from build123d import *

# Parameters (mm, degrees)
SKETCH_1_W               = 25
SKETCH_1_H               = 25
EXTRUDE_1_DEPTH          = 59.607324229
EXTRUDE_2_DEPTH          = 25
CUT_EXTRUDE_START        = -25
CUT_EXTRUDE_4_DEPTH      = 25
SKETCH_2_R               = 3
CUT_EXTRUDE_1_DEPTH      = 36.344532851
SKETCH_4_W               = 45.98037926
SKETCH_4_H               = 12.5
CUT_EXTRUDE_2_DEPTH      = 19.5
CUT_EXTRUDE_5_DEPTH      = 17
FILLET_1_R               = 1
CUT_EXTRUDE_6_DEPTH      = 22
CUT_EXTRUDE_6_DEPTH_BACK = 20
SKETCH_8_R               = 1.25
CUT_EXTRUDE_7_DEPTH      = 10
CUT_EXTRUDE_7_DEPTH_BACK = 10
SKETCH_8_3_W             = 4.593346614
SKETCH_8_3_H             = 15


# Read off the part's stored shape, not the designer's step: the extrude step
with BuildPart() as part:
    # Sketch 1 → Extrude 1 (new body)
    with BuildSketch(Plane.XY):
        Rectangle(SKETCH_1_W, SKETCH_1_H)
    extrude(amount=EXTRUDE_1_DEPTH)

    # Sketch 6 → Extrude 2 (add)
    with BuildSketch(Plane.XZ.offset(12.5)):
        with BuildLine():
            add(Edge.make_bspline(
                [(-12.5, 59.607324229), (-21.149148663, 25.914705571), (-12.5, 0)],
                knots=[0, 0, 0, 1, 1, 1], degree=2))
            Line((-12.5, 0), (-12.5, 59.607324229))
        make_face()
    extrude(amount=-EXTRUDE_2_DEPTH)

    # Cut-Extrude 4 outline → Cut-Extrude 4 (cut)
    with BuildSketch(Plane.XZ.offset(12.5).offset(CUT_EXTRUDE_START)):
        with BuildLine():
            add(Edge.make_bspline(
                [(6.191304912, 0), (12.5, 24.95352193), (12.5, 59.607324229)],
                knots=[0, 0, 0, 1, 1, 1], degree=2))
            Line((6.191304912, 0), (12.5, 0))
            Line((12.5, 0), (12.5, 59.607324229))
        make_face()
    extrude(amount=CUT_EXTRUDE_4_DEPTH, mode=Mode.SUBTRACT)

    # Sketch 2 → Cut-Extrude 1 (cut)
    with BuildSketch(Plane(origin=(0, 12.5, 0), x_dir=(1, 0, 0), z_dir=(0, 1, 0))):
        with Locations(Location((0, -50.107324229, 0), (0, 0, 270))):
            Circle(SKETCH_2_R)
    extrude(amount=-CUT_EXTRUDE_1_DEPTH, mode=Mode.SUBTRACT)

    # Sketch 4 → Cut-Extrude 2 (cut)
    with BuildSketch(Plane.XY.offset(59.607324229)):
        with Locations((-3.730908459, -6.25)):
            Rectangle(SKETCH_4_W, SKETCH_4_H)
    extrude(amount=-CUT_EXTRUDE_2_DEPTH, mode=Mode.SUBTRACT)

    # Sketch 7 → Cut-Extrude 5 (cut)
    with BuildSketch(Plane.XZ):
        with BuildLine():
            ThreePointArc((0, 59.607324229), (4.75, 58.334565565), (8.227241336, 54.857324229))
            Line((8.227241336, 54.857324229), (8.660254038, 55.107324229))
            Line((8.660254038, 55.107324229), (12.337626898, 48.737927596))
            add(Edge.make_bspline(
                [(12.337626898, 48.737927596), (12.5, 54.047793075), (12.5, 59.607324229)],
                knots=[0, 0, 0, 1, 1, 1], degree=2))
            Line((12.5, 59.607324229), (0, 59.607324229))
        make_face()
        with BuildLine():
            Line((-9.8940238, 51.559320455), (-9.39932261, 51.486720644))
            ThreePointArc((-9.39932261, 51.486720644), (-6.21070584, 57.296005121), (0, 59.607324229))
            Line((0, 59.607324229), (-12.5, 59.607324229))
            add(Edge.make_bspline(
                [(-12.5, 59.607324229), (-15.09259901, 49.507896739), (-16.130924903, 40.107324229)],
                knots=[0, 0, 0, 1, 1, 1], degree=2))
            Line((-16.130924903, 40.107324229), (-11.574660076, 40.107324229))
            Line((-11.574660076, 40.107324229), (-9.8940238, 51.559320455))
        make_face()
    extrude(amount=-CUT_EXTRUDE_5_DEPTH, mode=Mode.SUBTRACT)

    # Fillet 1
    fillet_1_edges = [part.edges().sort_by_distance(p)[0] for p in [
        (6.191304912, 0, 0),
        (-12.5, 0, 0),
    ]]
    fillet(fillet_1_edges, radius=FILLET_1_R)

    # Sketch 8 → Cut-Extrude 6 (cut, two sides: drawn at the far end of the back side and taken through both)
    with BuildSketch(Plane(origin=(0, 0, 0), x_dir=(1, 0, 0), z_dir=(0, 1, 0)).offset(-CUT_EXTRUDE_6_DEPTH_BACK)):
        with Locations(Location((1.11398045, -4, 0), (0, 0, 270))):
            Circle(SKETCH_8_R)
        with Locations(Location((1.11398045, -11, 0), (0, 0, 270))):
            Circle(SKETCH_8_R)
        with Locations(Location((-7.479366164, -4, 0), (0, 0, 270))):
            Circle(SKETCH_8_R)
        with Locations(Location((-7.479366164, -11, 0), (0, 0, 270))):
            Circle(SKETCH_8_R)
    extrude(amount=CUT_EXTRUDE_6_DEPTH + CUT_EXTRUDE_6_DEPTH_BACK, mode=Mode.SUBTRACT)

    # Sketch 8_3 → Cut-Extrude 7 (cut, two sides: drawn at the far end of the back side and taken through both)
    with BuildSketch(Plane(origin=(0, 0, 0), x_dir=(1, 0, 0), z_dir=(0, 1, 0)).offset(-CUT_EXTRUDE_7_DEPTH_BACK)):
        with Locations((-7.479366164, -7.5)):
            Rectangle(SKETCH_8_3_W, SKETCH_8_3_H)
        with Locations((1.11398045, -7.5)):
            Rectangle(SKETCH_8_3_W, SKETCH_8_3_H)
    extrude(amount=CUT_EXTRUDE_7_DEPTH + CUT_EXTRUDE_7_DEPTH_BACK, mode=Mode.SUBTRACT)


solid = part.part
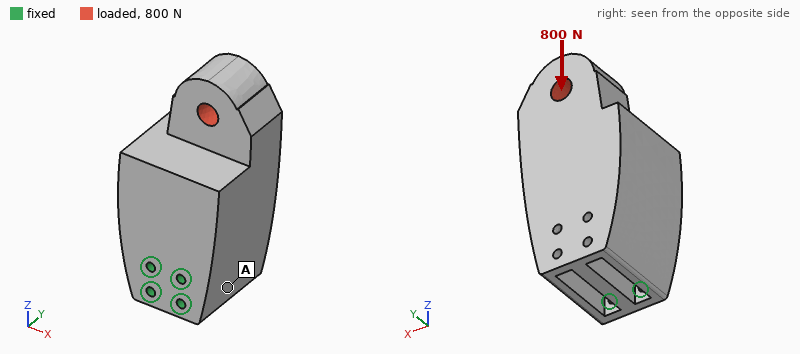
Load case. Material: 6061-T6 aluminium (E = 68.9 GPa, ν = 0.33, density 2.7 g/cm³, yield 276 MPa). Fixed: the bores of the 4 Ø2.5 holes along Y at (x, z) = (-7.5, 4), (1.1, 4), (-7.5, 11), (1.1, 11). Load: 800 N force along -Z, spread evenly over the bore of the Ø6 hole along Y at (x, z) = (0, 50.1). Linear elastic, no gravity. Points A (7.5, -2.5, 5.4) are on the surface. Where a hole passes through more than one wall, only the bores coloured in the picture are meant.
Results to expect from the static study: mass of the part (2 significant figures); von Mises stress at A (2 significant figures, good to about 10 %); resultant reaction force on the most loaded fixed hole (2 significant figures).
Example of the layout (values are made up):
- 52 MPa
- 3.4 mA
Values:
- 73 g
- 12 MPa
- 800 N
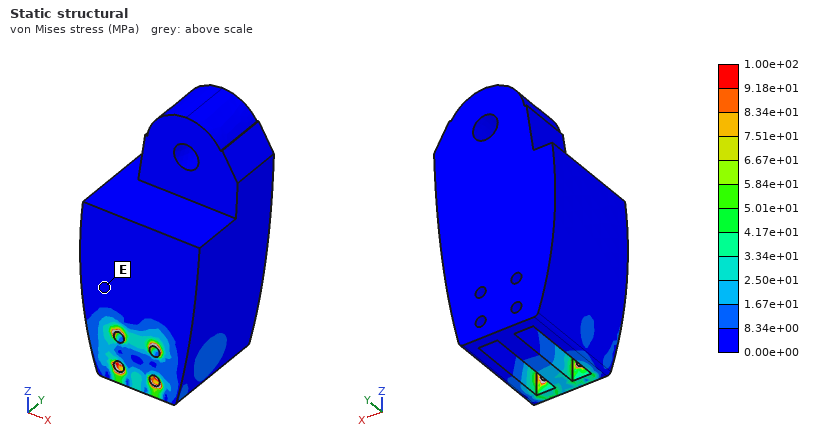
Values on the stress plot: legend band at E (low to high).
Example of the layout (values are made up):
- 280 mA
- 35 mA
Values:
- 0.00e+00 to 8.34e+00 MPa
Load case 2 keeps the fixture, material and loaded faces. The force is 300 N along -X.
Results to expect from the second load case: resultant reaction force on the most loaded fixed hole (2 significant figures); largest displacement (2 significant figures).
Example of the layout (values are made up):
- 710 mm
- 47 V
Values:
- 700 N
- 35 µm
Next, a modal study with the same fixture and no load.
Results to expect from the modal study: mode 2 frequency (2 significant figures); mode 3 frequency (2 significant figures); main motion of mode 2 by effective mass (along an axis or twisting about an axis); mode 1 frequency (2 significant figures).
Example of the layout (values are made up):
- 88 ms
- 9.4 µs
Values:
- 3100 Hz
- 5300 Hz
- along X
- 2100 Hz
